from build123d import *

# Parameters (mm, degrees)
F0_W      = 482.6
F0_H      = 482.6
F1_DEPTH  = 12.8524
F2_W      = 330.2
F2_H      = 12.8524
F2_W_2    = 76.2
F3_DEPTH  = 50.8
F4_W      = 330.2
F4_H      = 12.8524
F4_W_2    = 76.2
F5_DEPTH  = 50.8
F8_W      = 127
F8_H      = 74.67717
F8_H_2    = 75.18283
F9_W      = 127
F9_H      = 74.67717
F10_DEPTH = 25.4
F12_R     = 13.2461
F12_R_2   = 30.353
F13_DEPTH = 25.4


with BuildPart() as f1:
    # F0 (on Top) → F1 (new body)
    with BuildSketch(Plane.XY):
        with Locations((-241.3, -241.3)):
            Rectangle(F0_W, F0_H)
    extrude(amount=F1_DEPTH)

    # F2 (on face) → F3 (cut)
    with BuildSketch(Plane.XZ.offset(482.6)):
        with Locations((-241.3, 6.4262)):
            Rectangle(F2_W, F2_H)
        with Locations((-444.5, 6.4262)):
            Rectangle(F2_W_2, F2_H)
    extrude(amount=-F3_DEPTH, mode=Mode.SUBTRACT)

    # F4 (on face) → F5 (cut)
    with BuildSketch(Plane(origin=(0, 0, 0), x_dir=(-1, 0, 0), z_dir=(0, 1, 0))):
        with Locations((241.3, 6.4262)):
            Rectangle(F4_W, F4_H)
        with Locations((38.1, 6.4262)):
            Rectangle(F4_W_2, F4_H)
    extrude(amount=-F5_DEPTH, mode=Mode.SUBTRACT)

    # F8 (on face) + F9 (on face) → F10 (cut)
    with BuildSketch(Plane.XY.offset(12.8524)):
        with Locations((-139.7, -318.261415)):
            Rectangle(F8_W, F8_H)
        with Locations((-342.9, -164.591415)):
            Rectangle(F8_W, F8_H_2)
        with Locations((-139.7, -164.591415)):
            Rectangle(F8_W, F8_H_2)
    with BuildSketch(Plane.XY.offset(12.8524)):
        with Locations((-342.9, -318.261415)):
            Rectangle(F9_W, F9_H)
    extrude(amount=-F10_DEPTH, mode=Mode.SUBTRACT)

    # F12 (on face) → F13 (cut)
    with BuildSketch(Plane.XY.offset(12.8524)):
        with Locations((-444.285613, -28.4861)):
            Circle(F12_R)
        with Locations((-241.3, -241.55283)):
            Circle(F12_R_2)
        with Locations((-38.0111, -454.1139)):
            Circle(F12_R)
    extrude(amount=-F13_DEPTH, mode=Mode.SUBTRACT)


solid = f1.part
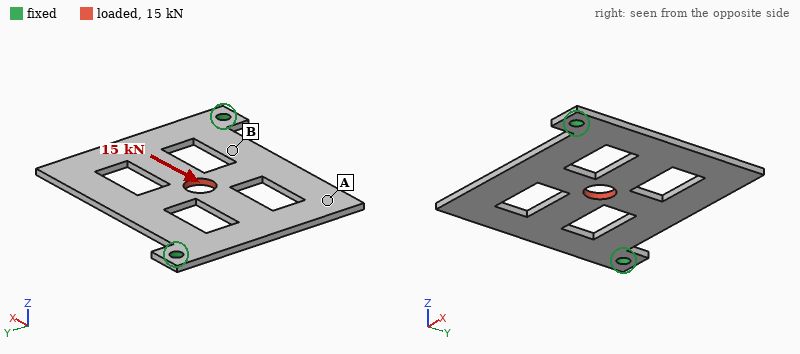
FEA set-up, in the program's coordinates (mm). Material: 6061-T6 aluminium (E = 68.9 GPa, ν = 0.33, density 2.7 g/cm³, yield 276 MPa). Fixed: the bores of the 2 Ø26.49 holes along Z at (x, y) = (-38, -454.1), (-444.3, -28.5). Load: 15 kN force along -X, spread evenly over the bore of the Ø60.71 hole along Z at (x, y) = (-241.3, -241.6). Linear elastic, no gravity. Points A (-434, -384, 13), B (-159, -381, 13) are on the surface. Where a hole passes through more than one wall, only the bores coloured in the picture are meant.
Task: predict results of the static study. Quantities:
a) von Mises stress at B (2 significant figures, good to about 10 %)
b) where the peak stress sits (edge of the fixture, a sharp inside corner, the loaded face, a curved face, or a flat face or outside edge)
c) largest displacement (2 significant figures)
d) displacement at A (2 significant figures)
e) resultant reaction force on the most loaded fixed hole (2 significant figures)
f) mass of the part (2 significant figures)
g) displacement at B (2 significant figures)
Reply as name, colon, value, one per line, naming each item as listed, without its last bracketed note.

von Mises stress at B: 7.6 MPa
where the peak stress sits: edge of the fixture
largest displacement: 84 µm
displacement at A: 50 µm
resultant reaction force on the most loaded fixed hole: 7.5 kN
mass of the part: 5.2 kg
displacement at B: 41 µm
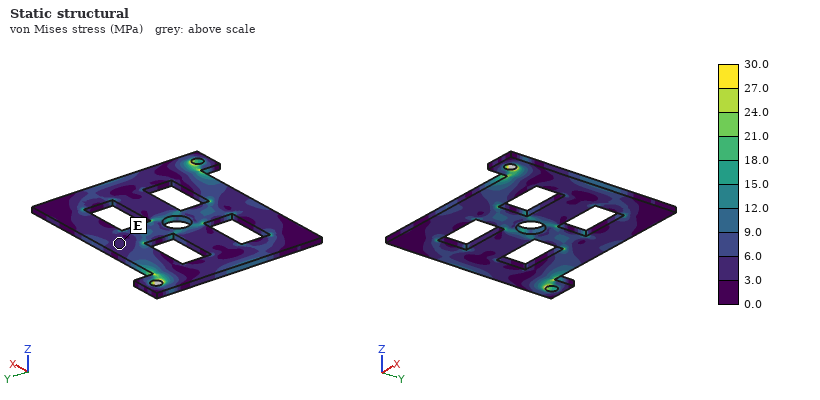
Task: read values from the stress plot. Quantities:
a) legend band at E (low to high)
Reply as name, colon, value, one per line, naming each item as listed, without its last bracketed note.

legend band at E: 3.0 to 6.0 MPa
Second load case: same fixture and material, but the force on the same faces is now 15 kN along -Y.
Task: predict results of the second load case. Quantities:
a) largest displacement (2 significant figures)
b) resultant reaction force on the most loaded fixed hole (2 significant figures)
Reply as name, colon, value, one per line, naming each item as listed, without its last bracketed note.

largest displacement: 87 µm
resultant reaction force on the most loaded fixed hole: 7.5 kN
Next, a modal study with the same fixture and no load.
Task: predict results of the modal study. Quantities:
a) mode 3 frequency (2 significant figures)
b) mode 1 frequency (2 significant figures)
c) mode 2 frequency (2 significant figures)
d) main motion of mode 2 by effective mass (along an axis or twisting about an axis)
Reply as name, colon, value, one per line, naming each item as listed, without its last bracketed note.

mode 3 frequency: 280 Hz
mode 1 frequency: 84 Hz
mode 2 frequency: 110 Hz
main motion of mode 2 by effective mass: along Z
